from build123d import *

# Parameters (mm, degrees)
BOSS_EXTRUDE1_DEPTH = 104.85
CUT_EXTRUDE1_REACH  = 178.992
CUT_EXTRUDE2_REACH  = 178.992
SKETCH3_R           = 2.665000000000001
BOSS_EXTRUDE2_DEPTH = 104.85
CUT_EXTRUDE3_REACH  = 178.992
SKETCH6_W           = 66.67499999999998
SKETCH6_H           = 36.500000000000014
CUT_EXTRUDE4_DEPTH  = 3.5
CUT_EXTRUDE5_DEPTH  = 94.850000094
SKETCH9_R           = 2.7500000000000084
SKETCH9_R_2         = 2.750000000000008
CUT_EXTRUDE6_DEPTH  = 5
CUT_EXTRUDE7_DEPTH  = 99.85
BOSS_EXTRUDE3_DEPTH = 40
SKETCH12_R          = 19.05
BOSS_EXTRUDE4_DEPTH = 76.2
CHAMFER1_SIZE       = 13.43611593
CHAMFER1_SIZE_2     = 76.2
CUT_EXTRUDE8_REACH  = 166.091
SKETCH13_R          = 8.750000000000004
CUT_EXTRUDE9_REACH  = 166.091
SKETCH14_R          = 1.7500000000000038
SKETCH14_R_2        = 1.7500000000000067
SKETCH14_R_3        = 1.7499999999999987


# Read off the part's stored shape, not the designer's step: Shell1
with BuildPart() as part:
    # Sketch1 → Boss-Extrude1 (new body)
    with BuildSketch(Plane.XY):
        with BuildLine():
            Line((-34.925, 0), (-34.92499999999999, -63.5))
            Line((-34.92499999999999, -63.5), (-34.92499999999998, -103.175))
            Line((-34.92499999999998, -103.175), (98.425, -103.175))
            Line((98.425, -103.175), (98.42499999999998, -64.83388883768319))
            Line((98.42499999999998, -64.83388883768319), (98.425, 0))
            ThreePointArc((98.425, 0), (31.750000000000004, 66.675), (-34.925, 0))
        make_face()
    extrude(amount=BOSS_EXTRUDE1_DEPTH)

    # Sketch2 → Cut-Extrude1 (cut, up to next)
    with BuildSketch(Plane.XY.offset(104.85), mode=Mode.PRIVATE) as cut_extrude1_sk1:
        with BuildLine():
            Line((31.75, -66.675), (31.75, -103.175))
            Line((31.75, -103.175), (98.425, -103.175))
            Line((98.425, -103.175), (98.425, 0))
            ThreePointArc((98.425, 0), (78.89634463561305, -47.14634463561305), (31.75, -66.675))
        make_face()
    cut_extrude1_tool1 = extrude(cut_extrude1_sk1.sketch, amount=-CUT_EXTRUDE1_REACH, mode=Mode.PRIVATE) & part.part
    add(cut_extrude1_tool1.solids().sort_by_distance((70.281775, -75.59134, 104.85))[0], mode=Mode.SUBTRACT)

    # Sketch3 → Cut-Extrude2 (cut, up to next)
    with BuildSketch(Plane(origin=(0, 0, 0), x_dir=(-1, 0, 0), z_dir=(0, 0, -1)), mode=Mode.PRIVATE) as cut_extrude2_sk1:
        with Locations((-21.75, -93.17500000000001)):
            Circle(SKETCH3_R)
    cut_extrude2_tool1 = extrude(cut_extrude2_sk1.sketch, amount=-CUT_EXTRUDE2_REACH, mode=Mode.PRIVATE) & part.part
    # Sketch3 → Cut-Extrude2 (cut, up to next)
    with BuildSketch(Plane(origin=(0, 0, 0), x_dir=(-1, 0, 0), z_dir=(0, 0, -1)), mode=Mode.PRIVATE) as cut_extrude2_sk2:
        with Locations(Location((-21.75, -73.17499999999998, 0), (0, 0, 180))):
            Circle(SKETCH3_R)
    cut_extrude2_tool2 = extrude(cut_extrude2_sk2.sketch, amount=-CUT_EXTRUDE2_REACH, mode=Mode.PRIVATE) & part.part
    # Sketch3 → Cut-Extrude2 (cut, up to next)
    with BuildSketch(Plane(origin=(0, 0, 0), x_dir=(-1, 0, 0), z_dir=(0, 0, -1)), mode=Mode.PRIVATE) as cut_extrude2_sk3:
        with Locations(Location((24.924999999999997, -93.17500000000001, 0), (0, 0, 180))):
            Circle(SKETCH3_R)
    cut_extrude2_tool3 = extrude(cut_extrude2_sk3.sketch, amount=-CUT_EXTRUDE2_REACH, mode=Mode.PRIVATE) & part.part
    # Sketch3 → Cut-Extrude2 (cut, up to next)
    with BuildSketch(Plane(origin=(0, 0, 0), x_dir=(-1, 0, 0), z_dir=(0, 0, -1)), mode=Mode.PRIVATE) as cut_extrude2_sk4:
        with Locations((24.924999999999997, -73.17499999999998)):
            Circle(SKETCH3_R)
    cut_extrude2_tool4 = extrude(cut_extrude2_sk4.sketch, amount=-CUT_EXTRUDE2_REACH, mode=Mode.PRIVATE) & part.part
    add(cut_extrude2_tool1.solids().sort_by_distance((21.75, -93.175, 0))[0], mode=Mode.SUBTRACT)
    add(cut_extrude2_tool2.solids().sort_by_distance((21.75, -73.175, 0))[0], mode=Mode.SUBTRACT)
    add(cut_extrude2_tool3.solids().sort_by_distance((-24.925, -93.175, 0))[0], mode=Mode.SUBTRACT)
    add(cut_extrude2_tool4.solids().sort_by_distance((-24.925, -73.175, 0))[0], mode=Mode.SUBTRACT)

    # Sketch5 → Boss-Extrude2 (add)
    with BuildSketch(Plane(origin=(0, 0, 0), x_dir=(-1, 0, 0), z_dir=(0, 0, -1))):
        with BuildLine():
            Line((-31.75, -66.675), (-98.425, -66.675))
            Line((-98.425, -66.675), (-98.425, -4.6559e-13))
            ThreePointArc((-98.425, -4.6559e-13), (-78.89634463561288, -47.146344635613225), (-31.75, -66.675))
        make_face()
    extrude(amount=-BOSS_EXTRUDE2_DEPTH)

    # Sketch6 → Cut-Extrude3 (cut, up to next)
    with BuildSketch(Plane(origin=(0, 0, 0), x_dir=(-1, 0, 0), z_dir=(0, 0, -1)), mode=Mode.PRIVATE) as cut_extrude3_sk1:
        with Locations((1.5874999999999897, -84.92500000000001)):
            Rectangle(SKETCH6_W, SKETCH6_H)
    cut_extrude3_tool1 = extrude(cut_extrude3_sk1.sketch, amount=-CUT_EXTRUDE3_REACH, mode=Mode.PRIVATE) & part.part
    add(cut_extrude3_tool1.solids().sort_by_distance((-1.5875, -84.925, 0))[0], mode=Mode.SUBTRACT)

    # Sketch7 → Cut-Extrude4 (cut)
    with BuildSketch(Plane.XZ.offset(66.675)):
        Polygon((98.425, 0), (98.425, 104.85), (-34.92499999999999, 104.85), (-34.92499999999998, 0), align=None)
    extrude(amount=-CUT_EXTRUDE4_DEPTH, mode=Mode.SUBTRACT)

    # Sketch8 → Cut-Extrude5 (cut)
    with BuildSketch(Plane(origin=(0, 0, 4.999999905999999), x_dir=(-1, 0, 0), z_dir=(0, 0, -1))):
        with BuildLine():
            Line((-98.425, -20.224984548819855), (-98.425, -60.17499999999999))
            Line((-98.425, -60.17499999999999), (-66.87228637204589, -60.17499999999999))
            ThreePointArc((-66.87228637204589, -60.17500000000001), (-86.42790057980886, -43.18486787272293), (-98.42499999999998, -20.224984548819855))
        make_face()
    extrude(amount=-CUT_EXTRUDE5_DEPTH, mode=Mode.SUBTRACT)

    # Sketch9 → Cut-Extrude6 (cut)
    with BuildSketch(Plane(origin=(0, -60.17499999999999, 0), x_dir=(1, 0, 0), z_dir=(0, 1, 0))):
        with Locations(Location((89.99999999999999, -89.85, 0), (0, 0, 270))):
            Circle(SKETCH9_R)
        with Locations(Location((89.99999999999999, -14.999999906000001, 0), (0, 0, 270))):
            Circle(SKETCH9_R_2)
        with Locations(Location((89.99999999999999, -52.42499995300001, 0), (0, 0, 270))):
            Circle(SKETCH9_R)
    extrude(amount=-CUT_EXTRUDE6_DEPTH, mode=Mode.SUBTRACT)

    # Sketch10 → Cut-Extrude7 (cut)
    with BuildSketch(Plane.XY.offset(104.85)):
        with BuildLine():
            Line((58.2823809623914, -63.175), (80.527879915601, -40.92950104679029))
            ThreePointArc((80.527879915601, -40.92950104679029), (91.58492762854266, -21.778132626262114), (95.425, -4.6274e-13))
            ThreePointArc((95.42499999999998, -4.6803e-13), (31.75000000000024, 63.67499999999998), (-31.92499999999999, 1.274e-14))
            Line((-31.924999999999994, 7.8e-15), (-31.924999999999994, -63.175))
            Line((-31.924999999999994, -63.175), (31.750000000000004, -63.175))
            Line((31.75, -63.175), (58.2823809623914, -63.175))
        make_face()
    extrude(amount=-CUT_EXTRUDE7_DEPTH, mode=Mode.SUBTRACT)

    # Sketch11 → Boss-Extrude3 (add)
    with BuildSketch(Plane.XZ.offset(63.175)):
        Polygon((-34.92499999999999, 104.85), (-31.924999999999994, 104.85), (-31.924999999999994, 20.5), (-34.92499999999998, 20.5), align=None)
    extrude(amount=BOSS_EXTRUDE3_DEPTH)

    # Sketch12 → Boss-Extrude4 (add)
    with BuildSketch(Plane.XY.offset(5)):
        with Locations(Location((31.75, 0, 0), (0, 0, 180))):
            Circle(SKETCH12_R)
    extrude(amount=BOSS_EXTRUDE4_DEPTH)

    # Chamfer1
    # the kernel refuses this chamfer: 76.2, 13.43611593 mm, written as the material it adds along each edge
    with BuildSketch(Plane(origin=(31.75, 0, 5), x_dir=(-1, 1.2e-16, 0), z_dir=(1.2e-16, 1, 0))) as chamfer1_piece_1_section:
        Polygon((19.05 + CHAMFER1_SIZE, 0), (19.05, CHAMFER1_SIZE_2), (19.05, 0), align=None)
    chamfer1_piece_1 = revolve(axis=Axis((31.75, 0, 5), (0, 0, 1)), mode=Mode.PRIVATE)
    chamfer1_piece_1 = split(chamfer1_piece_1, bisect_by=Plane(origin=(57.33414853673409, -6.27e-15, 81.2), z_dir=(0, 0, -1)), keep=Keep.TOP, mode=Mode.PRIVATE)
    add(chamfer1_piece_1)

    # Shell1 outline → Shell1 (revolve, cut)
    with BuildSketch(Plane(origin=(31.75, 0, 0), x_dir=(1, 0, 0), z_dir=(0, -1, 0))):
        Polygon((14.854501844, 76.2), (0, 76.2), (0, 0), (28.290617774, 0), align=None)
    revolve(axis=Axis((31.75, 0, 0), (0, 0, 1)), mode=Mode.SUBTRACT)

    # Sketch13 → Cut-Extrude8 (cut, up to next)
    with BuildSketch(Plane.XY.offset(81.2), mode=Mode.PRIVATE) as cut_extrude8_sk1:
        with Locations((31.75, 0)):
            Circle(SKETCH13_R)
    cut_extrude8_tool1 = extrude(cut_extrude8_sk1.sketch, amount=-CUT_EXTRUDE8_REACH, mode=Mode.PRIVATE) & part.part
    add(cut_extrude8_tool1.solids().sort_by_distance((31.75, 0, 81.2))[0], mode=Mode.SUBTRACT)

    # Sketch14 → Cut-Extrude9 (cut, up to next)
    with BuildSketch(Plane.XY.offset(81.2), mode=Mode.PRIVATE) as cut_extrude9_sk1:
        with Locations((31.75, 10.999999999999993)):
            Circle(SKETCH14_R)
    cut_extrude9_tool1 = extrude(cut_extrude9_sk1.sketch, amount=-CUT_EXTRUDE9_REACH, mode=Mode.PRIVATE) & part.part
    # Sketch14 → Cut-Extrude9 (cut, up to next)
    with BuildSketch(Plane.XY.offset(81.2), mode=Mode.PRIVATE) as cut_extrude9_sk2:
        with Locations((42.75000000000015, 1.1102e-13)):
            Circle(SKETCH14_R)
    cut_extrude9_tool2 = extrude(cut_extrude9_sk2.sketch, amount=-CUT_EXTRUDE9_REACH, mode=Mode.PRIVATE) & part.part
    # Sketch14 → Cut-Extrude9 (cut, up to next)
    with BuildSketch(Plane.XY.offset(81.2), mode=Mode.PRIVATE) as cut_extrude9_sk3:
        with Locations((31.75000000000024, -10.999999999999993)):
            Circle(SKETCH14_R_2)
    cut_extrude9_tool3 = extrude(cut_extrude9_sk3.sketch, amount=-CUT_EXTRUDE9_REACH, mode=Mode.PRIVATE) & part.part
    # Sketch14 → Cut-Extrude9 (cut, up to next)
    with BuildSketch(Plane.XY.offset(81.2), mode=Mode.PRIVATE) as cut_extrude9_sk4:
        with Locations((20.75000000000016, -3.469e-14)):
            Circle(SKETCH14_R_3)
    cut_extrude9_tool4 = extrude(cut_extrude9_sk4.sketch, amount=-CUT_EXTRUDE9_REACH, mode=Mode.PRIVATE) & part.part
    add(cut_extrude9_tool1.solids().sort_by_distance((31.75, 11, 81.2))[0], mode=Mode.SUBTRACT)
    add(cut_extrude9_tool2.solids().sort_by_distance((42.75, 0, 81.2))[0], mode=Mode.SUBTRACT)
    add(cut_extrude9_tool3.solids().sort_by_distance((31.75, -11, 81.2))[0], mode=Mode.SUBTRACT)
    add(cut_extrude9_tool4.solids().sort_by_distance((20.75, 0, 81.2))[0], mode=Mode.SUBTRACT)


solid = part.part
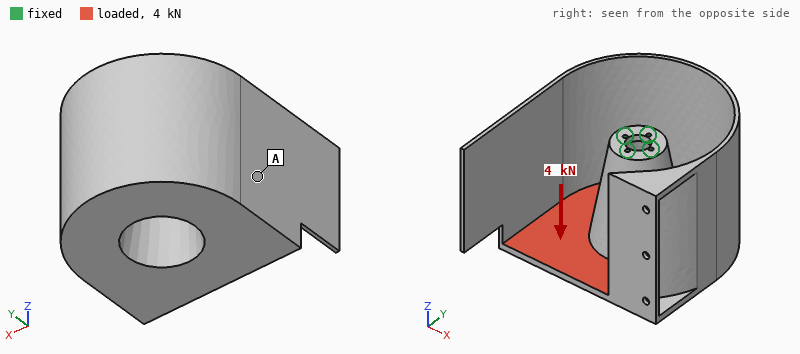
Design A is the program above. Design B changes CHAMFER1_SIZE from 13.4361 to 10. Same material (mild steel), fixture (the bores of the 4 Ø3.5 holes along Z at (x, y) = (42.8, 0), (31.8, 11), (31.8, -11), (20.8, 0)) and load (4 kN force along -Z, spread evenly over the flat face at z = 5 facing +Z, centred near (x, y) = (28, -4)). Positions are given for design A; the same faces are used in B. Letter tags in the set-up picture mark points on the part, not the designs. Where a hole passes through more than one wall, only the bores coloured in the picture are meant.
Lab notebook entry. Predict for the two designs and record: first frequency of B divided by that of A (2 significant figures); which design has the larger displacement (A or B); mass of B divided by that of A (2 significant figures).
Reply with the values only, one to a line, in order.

0.95
B
0.92
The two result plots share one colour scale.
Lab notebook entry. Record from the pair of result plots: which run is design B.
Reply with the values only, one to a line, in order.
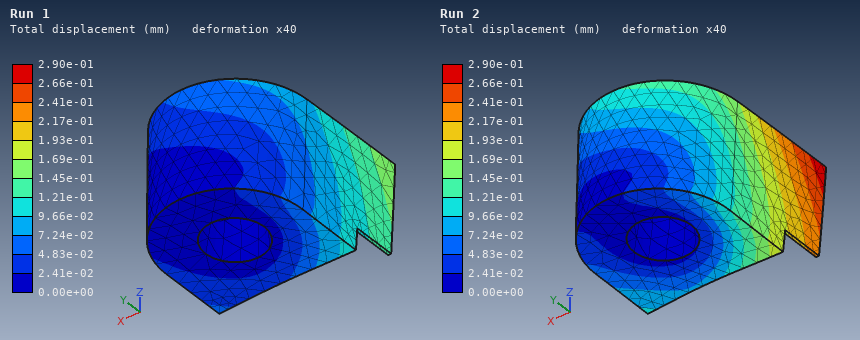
Run 2
